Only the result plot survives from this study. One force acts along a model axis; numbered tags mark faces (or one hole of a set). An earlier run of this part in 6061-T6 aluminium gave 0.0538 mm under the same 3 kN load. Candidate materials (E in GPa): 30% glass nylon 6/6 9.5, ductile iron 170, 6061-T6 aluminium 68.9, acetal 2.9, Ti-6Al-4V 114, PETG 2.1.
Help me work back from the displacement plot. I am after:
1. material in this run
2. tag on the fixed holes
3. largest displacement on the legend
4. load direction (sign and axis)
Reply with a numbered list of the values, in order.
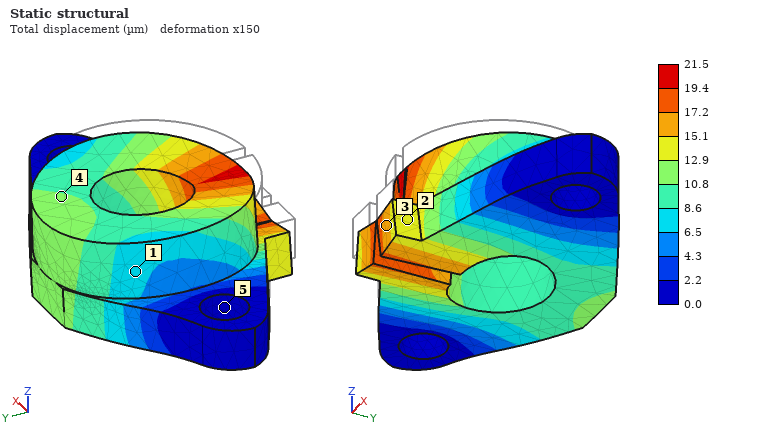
1. ductile iron
2. 5
3. 21.5 µm
4. -Z
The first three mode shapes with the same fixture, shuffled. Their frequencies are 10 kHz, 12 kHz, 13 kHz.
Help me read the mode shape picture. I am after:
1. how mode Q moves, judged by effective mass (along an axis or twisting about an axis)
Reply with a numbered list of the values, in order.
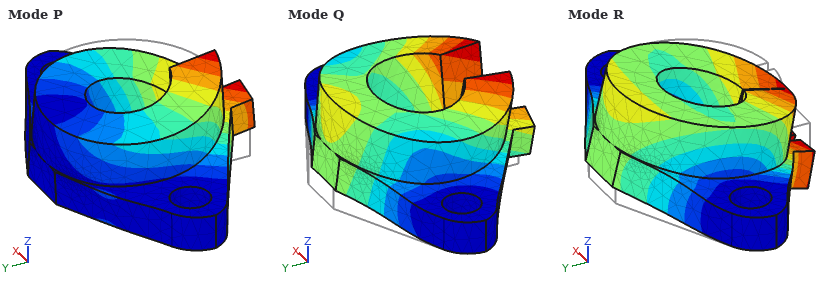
1. along Z
